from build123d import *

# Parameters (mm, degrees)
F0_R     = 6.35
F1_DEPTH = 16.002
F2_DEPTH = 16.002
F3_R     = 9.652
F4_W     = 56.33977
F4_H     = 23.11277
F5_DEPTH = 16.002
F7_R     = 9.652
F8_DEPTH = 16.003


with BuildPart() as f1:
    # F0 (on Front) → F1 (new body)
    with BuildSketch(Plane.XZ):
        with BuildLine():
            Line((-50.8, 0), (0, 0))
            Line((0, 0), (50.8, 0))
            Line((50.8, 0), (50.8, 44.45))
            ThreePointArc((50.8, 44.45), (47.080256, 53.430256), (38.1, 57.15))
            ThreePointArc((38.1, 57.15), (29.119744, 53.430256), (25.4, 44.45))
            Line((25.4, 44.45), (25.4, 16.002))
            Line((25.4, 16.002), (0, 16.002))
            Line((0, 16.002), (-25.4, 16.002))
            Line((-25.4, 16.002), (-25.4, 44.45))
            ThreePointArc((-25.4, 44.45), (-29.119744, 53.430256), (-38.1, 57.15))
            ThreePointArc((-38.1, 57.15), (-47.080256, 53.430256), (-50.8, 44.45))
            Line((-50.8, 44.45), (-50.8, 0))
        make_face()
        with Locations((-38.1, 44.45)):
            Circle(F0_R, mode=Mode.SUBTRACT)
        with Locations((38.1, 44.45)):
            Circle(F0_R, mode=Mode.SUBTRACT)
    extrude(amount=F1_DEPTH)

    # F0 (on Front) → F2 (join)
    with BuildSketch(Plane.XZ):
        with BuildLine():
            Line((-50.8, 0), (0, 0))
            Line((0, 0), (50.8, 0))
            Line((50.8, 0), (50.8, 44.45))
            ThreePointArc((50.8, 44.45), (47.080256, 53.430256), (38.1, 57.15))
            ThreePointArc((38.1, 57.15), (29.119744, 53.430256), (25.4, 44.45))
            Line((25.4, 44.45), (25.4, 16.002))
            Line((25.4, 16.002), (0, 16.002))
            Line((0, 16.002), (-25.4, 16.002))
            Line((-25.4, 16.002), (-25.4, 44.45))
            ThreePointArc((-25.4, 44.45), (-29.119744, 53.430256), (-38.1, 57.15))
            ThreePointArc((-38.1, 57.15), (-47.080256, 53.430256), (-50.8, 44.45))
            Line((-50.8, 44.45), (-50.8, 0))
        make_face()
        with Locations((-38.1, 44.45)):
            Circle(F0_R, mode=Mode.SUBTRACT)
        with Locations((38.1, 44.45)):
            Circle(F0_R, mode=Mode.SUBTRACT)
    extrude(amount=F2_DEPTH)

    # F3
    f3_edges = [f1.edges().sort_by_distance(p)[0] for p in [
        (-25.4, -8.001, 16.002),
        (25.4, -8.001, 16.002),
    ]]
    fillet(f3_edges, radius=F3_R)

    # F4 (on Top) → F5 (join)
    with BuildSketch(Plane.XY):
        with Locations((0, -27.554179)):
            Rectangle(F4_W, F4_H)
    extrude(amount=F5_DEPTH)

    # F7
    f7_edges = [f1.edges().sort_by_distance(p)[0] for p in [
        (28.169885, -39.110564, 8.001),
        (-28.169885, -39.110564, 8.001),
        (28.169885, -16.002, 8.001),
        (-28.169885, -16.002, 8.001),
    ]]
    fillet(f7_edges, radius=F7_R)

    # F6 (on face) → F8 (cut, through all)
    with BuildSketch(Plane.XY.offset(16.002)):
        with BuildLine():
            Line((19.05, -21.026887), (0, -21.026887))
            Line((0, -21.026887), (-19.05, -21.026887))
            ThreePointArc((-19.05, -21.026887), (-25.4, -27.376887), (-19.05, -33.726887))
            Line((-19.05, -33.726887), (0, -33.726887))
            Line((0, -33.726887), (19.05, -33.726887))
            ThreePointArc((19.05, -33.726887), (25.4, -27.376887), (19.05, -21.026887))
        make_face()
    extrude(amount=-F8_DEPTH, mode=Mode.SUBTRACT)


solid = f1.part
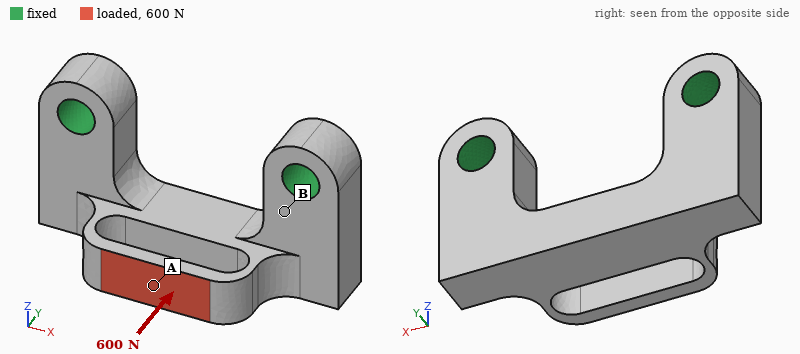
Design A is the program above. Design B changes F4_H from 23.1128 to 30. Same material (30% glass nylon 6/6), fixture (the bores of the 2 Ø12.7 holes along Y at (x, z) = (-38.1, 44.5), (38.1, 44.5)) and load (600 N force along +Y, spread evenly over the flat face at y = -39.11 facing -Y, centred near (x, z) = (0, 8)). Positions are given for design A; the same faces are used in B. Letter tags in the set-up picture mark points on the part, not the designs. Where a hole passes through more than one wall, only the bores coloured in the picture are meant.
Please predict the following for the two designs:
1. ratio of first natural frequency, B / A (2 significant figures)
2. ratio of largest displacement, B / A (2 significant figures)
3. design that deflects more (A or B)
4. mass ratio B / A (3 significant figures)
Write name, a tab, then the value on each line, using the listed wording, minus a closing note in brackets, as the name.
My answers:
ratio of first natural frequency, B / A	0.90
ratio of largest displacement, B / A	0.54
design that deflects more	A
mass ratio B / A	1.05
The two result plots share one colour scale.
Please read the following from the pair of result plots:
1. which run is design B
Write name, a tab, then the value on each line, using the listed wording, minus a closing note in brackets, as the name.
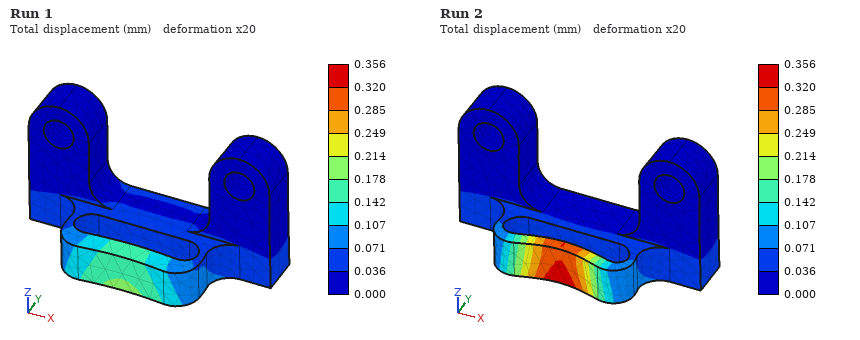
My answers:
which run is design B	Run 1
